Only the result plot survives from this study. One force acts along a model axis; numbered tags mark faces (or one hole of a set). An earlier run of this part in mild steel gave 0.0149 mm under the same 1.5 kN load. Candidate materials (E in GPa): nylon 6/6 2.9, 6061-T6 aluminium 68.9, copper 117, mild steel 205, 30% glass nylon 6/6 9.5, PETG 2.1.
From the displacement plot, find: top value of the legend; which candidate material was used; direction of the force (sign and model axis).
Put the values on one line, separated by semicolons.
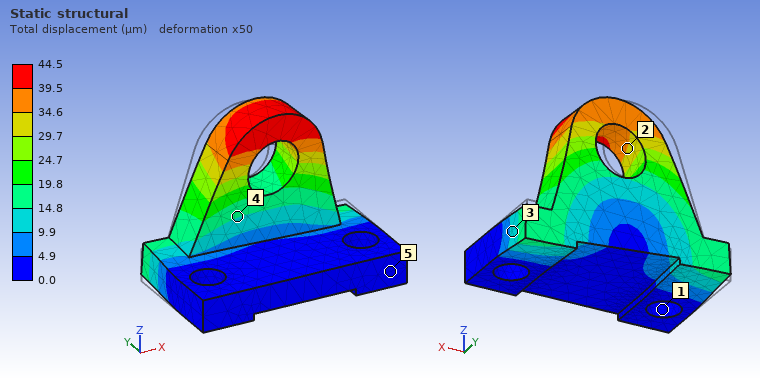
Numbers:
44.5 µm; 6061-T6 aluminium; +X
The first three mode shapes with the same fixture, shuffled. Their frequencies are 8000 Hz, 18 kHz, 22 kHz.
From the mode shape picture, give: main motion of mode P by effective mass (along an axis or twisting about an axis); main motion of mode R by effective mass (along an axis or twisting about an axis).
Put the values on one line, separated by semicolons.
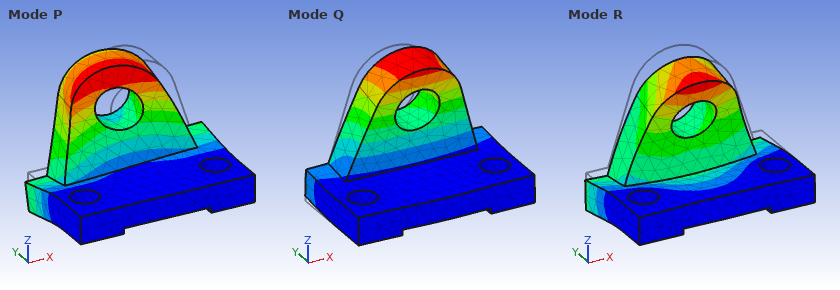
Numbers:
along X; along Z
